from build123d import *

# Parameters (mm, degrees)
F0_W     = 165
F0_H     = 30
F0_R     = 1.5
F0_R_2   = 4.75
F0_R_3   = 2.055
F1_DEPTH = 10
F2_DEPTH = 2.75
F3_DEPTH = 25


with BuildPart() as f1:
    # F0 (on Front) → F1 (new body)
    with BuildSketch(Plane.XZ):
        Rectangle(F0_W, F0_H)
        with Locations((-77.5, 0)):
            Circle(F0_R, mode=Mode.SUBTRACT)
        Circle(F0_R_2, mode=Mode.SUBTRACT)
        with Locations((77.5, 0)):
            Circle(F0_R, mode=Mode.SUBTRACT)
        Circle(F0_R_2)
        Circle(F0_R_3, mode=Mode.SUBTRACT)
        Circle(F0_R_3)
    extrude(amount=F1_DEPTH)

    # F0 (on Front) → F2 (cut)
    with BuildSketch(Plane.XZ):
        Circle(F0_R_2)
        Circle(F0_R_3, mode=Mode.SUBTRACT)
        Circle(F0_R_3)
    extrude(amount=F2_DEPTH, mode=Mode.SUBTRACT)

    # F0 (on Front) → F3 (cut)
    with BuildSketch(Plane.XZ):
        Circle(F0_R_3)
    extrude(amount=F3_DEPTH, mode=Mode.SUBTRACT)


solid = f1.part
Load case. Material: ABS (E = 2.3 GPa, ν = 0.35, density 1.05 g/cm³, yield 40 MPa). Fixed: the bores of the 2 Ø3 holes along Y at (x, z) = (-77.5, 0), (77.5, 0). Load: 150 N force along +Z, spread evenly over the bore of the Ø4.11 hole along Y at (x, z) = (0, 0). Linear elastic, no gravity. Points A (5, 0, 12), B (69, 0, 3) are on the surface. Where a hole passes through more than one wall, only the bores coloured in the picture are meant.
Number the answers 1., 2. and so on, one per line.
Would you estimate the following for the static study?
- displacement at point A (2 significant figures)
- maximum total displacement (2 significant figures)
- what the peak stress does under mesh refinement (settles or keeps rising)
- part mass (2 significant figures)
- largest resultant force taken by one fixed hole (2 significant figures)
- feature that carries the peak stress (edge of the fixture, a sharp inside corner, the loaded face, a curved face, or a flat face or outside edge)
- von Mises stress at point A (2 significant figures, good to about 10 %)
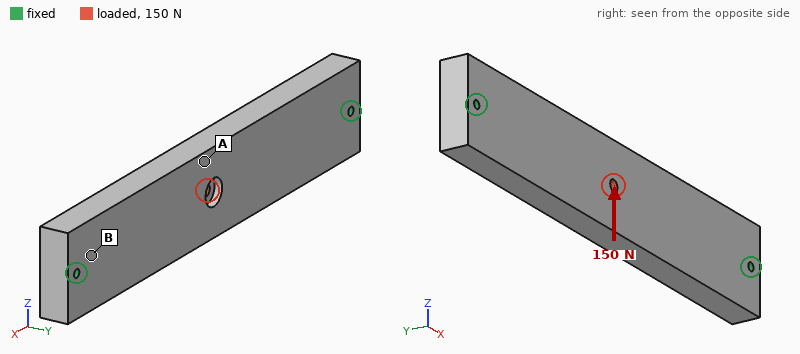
1. 0.20 mm
2. 0.22 mm
3. keeps rising
4. 52 g
5. 75 N
6. edge of the fixture
7. 2.6 MPa
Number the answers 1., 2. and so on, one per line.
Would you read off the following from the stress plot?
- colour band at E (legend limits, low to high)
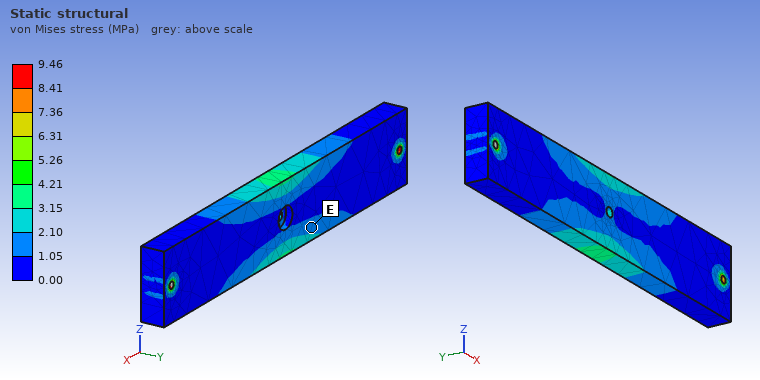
1. 1.05 to 2.10 MPa
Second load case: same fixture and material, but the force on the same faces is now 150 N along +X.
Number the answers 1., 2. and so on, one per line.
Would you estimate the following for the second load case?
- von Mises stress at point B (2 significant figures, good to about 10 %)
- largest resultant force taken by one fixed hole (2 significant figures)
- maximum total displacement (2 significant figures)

1. 0.52 MPa
2. 75 N
3. 15 µm
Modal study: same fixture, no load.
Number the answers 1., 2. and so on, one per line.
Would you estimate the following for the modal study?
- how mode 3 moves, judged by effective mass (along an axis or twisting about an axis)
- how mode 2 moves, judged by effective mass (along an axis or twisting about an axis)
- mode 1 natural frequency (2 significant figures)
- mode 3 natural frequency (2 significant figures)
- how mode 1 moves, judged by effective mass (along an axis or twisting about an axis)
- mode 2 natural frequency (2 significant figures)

1. twisting about Z
2. along Z
3. 530 Hz
4. 1500 Hz
5. along Y
6. 890 Hz
